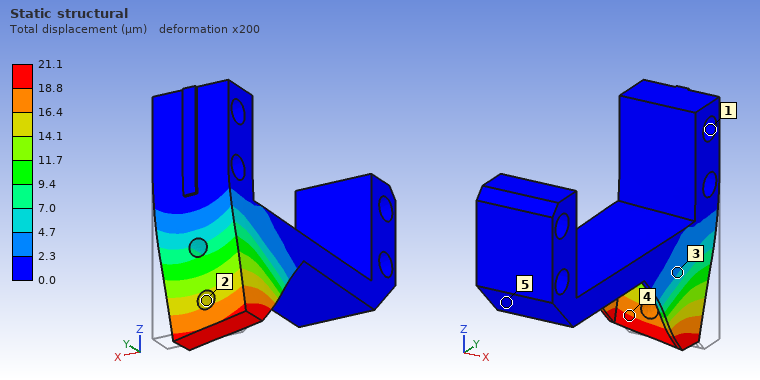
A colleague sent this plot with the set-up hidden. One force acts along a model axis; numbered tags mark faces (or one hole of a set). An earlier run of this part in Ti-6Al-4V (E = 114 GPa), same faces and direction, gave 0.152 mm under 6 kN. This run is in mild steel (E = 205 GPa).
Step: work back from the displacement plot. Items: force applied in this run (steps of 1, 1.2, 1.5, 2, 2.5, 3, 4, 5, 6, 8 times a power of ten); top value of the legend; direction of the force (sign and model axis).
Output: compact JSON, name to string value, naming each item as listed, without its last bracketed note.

{"force applied in this run": "1.5 kN", "top value of the legend": "21.1 µm", "direction of the force": "-X"}
